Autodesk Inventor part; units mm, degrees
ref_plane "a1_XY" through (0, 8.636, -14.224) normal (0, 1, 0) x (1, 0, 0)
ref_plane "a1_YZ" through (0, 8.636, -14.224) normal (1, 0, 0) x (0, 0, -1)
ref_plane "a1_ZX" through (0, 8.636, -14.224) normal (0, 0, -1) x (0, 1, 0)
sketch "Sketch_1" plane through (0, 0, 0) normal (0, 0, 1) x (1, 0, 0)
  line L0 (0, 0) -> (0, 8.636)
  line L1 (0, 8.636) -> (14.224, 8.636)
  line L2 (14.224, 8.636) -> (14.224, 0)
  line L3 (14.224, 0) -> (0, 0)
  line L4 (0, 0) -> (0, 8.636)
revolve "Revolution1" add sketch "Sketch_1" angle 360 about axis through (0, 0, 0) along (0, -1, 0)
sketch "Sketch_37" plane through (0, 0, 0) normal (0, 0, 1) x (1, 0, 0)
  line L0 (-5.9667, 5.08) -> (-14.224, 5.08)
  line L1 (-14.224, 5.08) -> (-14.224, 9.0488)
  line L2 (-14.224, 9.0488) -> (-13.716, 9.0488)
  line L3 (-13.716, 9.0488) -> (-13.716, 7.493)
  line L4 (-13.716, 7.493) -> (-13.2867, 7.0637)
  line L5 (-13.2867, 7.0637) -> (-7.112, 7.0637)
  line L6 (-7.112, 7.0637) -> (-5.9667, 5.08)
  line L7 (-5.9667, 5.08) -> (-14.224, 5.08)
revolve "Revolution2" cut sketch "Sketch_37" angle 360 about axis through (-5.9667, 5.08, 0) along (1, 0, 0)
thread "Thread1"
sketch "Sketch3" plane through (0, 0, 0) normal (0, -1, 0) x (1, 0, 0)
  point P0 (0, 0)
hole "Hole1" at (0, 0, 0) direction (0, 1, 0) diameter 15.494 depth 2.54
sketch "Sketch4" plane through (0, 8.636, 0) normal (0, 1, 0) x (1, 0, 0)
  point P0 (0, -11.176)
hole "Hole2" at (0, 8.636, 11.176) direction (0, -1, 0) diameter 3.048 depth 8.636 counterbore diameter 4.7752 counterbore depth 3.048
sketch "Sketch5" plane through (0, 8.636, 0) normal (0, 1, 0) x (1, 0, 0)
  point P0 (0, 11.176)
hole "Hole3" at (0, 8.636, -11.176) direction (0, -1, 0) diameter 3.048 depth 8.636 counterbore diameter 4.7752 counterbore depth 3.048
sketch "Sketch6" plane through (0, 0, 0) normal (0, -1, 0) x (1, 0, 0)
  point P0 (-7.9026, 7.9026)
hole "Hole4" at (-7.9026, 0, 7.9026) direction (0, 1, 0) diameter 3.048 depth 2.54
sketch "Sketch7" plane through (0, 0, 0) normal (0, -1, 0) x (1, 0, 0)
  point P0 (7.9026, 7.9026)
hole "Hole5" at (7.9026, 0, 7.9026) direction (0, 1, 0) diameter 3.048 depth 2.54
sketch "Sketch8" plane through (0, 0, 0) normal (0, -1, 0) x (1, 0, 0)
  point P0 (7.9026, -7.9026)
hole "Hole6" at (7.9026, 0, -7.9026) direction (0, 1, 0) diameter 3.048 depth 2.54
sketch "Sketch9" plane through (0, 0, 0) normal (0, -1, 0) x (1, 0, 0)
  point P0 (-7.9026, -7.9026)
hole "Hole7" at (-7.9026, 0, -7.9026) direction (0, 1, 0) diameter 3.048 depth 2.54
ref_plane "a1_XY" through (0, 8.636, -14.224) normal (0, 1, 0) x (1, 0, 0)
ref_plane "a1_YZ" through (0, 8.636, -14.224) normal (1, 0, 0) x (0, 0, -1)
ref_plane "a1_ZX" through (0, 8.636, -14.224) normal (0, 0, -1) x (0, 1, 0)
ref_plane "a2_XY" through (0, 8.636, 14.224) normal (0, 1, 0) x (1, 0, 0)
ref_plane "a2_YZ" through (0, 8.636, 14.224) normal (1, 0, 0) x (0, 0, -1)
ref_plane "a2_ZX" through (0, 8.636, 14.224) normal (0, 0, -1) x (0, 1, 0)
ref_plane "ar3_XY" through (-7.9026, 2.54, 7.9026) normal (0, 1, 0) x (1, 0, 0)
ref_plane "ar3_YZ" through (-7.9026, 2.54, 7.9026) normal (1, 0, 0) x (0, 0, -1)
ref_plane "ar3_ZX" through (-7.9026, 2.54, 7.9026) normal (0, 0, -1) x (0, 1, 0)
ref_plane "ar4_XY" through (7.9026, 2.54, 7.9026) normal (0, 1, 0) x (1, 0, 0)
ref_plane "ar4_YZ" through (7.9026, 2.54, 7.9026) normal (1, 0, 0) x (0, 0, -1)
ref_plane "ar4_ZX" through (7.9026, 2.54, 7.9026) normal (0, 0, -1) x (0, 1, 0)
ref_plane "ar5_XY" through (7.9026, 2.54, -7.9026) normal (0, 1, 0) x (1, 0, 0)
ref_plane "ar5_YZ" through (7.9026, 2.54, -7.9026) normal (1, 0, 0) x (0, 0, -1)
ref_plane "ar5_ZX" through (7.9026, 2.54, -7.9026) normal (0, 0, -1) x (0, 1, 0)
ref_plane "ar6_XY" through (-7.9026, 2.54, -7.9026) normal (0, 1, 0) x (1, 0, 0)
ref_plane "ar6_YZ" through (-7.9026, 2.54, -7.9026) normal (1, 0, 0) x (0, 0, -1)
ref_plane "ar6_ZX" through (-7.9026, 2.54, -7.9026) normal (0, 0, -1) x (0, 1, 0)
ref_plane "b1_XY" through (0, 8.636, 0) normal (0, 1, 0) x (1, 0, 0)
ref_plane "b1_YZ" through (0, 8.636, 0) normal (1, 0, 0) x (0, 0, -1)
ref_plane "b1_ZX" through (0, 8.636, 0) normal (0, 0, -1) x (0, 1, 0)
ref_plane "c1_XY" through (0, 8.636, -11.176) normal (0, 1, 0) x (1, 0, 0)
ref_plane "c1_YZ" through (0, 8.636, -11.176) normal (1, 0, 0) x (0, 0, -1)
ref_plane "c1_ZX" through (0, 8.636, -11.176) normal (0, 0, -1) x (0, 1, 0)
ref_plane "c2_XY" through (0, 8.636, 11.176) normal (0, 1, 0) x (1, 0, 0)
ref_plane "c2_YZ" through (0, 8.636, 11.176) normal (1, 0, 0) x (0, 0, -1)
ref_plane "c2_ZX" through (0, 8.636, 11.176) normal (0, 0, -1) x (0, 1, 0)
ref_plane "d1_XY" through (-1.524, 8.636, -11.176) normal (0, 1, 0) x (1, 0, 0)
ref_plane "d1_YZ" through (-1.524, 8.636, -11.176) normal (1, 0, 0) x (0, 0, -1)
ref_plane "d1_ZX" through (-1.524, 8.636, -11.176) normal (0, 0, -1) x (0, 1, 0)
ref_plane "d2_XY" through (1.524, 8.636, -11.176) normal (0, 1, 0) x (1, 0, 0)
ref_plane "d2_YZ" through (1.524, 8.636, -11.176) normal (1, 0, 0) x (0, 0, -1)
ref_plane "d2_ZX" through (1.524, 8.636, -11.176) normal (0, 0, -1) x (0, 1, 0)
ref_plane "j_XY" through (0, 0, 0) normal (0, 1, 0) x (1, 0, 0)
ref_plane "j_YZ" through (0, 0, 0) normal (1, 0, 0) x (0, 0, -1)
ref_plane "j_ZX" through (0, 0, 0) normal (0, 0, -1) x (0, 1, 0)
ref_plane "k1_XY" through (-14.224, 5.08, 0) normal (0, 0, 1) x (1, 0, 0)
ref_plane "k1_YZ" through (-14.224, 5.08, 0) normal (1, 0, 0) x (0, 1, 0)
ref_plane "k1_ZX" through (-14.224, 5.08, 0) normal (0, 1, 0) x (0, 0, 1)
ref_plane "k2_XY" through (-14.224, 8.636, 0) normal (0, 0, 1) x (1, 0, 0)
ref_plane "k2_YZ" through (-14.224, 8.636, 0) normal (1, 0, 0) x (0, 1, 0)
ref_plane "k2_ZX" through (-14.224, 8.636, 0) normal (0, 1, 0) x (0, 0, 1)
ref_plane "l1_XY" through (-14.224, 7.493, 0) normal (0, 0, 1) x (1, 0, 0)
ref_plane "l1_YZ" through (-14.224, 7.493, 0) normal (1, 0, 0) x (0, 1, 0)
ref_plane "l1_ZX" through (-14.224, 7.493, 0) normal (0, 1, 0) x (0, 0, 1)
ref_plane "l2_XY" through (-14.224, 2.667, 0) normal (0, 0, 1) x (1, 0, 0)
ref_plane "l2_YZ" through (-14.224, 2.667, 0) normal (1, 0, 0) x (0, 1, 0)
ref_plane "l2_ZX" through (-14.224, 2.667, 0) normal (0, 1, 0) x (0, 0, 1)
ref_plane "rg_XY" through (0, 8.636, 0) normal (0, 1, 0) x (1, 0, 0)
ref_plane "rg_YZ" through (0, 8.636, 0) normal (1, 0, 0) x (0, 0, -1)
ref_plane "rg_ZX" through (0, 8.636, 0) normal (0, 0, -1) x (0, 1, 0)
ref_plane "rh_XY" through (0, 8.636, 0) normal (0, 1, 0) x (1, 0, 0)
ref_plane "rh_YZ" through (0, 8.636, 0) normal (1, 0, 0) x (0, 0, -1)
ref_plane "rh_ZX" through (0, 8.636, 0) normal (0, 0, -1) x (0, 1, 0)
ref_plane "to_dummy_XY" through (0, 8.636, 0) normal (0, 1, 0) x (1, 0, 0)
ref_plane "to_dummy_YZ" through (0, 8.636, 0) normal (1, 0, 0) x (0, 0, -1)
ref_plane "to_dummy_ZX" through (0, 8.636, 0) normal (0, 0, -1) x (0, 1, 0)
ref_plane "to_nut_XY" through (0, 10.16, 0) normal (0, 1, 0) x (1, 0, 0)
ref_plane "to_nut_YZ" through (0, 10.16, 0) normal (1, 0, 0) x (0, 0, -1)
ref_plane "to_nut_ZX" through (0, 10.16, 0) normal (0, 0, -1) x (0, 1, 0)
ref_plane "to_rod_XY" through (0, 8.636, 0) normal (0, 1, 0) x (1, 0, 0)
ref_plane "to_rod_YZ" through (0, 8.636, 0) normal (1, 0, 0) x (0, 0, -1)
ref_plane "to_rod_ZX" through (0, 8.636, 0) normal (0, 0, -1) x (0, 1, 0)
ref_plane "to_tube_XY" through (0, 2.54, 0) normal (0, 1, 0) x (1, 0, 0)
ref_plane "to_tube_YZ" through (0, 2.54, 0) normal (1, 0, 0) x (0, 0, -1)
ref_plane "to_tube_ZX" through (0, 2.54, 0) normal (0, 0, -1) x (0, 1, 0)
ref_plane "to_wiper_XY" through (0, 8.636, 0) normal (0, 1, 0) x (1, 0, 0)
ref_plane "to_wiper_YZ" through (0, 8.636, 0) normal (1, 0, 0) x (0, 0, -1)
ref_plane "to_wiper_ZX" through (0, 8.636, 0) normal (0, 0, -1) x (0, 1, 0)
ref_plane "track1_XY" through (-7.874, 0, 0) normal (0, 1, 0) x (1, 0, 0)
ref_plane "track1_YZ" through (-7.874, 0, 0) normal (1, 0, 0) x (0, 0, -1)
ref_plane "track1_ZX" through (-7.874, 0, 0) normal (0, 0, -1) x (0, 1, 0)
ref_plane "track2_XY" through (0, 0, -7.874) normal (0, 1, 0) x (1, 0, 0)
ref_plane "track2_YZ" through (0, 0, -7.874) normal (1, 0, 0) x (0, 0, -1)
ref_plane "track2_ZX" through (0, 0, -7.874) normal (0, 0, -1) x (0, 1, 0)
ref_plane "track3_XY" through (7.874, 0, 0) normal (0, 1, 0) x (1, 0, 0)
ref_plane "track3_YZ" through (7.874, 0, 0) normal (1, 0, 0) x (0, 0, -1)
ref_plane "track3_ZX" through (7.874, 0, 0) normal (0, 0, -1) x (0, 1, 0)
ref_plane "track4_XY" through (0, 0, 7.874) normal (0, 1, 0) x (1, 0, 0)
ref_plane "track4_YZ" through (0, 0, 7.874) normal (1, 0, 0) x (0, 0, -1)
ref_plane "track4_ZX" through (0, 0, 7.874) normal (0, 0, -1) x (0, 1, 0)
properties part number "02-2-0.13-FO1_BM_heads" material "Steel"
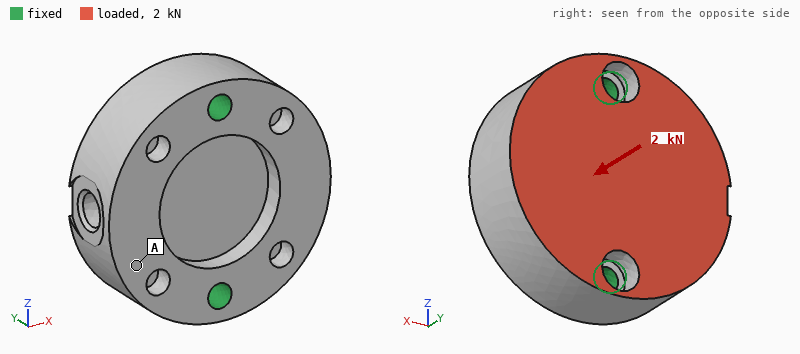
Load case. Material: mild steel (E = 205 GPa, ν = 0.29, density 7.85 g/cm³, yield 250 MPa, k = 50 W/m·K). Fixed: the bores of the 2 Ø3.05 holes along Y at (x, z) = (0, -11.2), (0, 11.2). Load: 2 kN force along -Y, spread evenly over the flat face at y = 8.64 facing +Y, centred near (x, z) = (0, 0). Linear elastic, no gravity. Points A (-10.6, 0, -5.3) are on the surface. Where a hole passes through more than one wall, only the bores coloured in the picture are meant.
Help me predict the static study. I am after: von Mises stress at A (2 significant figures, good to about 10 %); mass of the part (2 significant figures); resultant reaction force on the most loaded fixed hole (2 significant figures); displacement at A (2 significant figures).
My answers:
8.3 MPa
36 g
1.1 kN
2.5 µm
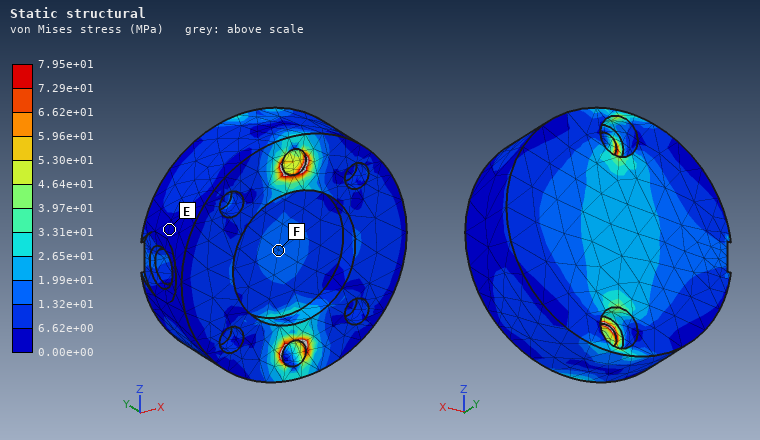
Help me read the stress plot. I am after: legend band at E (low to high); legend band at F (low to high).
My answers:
0.00e+00 to 6.62e+00 MPa
1.32e+01 to 1.99e+01 MPa
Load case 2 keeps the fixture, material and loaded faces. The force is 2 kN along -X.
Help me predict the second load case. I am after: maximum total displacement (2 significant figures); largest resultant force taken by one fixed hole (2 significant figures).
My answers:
7.5 µm
1.0 kN
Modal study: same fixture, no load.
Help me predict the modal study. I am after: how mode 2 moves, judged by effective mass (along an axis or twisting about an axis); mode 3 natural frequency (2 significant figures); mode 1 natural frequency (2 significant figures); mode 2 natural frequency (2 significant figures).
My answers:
along Y
42 kHz
17 kHz
26 kHz
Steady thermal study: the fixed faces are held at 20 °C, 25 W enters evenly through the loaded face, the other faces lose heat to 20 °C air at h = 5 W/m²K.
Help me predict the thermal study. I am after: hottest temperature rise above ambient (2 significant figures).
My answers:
23 K
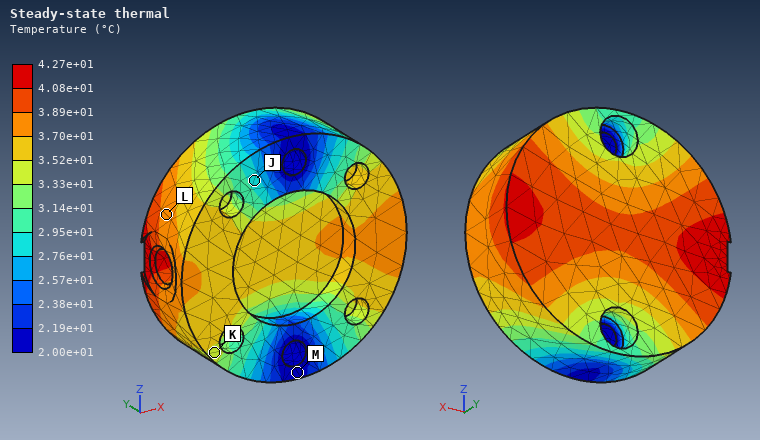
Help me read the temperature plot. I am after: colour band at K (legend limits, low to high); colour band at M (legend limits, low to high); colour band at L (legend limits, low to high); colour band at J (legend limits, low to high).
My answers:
3.33e+01 to 3.52e+01 °C
2.00e+01 to 2.19e+01 °C
3.70e+01 to 3.89e+01 °C
2.76e+01 to 2.95e+01 °C
